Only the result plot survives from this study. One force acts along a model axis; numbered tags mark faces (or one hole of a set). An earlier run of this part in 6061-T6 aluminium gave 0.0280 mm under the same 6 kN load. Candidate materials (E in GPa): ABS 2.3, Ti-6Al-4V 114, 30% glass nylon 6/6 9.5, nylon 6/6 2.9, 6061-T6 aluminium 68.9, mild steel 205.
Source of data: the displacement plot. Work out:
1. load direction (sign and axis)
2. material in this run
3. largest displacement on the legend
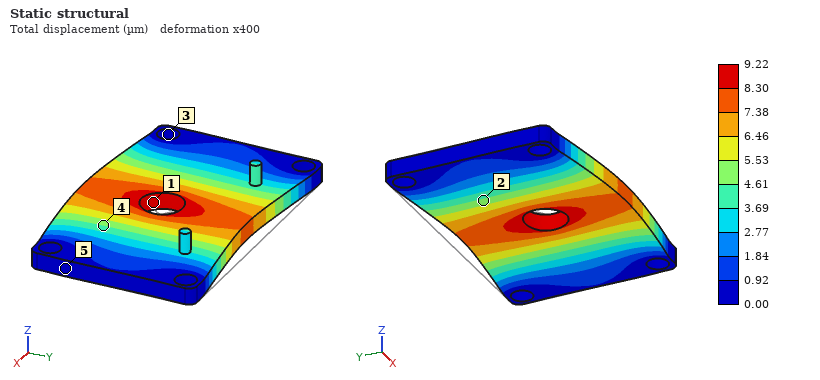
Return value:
-Y
mild steel
9.22 µm
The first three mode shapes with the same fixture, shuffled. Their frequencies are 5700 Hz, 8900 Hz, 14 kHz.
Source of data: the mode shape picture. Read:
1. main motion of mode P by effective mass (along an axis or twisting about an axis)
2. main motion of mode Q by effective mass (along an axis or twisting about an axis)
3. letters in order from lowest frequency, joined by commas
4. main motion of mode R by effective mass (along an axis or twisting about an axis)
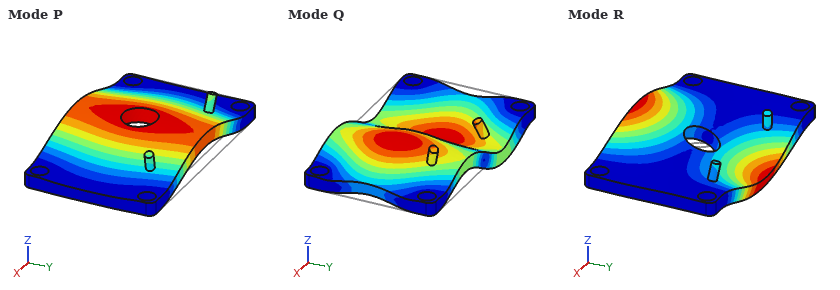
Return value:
along Z
twisting about Y
P, R, Q
twisting about X
